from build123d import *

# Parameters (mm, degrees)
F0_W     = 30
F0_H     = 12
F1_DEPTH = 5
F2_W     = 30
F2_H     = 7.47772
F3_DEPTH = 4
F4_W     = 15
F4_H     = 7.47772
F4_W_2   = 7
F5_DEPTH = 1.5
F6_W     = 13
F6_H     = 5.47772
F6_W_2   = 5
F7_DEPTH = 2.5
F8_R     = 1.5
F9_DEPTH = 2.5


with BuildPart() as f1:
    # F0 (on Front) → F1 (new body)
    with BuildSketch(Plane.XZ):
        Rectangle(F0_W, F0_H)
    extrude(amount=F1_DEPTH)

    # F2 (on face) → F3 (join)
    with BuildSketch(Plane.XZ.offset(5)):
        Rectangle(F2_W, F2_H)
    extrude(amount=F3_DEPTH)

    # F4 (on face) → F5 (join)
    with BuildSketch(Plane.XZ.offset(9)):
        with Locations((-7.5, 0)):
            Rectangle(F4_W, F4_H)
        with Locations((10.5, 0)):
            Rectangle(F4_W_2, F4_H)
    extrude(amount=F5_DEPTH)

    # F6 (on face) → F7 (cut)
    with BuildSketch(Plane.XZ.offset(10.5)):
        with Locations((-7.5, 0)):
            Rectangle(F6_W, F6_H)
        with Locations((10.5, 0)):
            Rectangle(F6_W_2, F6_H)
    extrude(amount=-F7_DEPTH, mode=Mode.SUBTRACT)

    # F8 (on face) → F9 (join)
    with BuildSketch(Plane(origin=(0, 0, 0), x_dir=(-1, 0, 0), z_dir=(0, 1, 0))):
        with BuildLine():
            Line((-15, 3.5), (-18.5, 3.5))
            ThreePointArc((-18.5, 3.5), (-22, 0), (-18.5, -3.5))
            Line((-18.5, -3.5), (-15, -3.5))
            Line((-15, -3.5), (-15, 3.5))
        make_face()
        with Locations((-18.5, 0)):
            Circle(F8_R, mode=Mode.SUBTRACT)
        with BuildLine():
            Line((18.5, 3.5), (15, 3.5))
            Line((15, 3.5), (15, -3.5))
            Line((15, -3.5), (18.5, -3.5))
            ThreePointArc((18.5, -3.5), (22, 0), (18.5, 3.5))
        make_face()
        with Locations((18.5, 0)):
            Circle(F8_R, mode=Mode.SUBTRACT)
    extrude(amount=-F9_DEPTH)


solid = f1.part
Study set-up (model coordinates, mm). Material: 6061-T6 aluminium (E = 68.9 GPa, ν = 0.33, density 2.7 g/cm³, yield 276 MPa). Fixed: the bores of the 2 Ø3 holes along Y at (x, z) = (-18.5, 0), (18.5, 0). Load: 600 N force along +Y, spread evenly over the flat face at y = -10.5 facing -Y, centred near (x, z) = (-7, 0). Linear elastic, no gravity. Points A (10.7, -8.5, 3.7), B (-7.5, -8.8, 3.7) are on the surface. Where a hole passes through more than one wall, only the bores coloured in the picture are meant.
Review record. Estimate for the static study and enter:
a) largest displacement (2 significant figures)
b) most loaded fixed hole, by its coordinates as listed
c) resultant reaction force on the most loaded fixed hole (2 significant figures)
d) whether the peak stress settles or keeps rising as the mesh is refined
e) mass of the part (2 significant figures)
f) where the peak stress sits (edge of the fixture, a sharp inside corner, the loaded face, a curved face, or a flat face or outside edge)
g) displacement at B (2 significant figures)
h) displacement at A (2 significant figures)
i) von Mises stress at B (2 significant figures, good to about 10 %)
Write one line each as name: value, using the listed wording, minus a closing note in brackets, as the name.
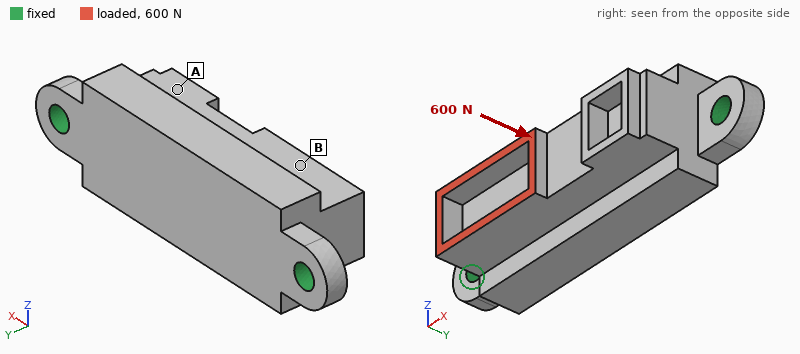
largest displacement: 11 µm
most loaded fixed hole, by its coordinates as listed: (-18.5, 0)
resultant reaction force on the most loaded fixed hole: 500 N
whether the peak stress settles or keeps rising as the mesh is refined: keeps rising
mass of the part: 7.8 g
where the peak stress sits: edge of the fixture
displacement at B: 11 µm
displacement at A: 5.6 µm
von Mises stress at B: 16 MPa
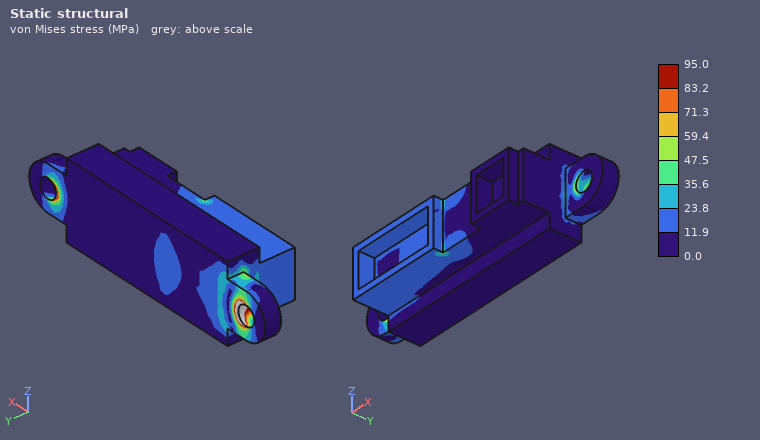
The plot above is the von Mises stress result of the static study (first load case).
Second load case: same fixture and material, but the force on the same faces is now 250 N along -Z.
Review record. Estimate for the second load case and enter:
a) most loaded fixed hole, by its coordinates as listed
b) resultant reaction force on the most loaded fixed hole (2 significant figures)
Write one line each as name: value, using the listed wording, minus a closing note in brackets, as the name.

most loaded fixed hole, by its coordinates as listed: (-18.5, 0)
resultant reaction force on the most loaded fixed hole: 180 N
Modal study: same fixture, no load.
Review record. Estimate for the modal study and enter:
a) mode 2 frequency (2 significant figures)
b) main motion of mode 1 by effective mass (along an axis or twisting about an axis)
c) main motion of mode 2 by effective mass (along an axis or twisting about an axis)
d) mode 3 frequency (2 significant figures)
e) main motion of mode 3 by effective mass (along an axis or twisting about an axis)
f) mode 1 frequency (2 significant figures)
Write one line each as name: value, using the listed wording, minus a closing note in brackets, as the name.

mode 2 frequency: 15 kHz
main motion of mode 1 by effective mass: along Z
main motion of mode 2 by effective mass: along Y
mode 3 frequency: 21 kHz
main motion of mode 3 by effective mass: along Z
mode 1 frequency: 8700 Hz
